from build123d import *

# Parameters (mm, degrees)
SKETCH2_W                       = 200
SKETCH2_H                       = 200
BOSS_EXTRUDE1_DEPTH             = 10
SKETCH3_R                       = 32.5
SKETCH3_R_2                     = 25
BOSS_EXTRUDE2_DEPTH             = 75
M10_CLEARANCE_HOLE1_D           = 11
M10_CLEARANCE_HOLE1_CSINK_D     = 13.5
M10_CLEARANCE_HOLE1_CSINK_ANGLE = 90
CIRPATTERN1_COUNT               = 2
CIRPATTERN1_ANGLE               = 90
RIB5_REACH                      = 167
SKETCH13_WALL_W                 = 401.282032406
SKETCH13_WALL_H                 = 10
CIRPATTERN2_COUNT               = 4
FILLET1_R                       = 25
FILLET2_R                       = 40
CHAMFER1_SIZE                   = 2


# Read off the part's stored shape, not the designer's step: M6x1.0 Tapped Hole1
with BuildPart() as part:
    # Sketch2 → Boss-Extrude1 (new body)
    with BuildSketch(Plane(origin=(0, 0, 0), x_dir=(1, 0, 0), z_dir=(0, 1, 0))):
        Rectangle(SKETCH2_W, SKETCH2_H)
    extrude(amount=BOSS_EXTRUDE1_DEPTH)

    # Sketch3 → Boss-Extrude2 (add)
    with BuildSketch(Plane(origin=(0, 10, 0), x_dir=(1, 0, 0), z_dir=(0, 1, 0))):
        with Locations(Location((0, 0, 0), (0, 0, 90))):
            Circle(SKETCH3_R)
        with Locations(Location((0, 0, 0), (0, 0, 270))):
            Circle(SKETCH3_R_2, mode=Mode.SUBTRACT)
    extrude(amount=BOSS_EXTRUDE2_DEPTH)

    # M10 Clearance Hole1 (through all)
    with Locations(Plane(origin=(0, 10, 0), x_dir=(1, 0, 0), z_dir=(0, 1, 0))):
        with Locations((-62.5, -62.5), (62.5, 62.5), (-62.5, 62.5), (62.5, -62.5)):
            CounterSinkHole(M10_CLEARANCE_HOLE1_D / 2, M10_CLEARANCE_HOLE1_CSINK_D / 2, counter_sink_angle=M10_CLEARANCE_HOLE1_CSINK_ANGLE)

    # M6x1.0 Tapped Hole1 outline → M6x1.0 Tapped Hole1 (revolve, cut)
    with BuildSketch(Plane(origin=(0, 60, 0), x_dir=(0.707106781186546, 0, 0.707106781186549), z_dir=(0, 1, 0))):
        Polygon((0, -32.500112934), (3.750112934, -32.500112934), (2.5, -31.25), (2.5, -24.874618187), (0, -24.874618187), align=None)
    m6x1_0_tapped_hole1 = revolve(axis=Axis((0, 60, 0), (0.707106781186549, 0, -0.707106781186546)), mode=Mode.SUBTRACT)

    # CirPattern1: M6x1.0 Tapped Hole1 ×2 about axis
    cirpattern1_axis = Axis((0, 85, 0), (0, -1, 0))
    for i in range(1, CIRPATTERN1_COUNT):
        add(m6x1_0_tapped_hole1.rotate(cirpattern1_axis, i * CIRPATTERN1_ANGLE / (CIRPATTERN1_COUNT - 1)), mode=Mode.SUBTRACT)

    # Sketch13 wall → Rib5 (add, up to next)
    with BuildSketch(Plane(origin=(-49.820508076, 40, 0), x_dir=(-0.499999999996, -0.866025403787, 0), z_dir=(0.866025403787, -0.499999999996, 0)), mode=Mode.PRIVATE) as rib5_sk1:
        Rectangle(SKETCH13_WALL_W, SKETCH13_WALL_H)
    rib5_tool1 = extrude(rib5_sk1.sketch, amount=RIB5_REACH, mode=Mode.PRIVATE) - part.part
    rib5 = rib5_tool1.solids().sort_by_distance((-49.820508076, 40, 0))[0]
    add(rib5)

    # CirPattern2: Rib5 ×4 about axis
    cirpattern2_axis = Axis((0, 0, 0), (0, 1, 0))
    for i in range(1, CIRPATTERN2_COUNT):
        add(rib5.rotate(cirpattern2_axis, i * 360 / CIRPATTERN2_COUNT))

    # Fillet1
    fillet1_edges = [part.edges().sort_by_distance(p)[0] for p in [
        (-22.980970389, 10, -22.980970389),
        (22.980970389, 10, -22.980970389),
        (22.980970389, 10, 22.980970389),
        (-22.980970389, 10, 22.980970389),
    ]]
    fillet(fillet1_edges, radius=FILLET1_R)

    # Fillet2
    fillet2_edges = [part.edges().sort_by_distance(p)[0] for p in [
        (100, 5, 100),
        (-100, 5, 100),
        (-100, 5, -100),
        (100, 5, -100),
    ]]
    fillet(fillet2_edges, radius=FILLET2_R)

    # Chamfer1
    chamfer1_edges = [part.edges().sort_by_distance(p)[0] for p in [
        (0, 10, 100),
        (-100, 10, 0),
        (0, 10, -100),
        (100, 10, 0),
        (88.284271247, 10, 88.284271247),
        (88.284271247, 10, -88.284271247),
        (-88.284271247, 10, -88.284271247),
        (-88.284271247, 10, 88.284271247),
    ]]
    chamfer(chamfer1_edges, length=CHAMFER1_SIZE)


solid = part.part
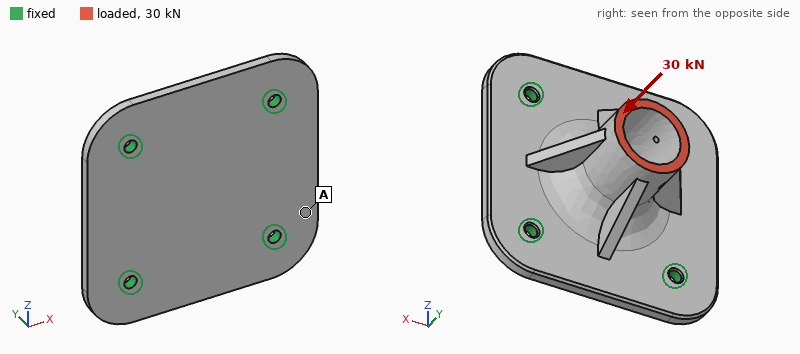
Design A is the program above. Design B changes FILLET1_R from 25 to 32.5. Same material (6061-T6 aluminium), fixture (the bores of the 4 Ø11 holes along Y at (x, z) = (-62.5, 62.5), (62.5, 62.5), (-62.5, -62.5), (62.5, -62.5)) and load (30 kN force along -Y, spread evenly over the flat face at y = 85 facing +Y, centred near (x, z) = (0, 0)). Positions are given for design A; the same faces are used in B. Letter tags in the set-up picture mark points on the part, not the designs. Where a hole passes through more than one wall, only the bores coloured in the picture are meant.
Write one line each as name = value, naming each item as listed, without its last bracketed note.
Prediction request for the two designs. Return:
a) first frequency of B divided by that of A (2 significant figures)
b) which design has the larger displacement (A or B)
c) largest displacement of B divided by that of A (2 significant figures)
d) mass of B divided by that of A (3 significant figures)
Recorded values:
first frequency of B divided by that of A = 1.0
which design has the larger displacement = A
largest displacement of B divided by that of A = 0.85
mass of B divided by that of A = 1.04
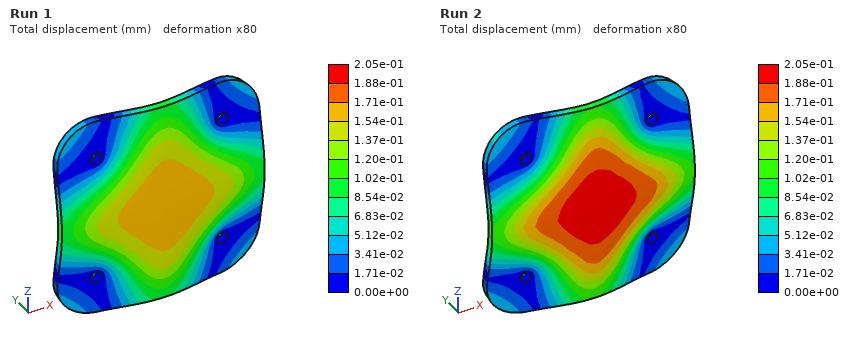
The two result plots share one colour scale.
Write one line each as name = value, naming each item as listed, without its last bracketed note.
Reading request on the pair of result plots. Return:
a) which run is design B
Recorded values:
which run is design B = Run 1
